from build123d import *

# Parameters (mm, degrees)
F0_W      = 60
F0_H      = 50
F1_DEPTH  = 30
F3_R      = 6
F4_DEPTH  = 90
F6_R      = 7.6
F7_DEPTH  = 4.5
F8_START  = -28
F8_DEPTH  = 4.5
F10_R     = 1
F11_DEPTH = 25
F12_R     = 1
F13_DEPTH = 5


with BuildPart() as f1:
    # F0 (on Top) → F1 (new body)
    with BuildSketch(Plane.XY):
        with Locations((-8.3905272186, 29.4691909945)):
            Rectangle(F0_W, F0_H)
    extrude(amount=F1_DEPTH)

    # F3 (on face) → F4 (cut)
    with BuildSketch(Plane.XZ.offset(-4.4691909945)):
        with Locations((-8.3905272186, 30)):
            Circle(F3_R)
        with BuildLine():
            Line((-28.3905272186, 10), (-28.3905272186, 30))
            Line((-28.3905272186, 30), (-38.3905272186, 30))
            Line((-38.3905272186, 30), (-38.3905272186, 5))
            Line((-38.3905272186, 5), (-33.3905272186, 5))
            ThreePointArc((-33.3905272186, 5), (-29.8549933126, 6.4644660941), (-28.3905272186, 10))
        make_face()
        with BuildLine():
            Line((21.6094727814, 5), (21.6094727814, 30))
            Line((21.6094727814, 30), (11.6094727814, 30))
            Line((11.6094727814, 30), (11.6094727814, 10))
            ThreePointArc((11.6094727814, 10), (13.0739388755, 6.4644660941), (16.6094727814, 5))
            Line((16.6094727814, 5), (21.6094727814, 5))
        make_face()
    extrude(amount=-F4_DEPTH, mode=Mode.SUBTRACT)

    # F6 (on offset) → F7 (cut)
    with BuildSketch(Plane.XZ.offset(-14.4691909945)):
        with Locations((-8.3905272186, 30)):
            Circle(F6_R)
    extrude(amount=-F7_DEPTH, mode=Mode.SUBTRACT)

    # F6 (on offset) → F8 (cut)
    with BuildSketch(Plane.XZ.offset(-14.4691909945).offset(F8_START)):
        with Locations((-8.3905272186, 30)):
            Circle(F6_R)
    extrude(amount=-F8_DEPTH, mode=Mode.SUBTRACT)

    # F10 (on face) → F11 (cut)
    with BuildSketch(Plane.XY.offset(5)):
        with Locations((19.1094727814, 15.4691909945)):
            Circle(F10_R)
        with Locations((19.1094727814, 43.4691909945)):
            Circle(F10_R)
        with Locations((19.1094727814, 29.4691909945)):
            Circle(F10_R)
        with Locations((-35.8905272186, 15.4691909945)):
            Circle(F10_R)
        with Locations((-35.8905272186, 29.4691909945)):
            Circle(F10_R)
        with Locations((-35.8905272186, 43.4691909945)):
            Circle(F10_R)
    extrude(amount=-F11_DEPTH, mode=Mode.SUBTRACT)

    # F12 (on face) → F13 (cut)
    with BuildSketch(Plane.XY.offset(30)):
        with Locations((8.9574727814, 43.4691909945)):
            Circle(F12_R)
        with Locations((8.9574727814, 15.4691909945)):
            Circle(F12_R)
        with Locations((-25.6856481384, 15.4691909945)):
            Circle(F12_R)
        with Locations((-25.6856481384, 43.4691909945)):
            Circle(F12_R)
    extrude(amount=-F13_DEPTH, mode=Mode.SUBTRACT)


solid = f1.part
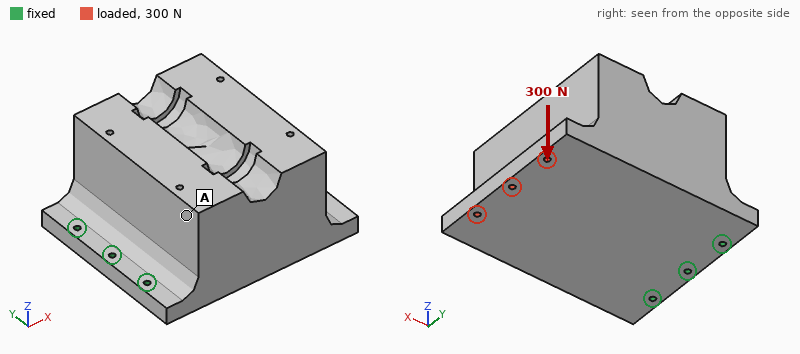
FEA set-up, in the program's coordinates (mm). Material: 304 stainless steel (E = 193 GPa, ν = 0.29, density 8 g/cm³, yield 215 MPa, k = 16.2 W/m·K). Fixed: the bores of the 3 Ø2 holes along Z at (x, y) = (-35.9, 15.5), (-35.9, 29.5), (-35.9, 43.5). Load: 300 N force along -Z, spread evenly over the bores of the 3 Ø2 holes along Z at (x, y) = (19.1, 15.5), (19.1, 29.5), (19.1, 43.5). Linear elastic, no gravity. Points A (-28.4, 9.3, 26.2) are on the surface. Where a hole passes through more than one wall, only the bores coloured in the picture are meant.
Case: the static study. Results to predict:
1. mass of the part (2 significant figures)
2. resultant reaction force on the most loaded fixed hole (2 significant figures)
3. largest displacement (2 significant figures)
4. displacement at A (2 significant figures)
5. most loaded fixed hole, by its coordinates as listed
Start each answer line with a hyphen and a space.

- 500 g
- 140 N
- 92 µm
- 39 µm
- (-35.9, 29.5)
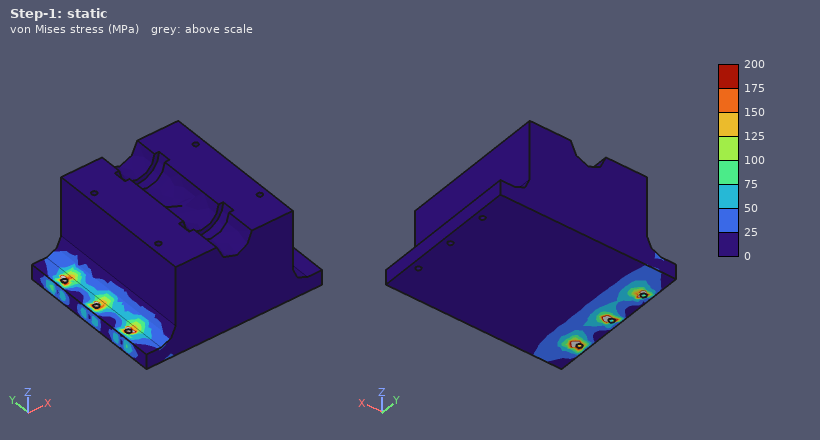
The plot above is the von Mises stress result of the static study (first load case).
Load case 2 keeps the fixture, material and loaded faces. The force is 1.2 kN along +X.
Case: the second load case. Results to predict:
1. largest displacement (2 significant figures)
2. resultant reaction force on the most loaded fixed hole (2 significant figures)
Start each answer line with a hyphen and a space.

- 3.9 µm
- 410 N
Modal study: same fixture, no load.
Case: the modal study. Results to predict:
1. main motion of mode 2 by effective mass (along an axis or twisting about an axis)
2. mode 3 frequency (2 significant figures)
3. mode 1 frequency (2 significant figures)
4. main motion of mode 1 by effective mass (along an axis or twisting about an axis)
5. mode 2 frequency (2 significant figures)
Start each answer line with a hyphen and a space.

- along Y
- 4000 Hz
- 700 Hz
- along Z
- 3200 Hz
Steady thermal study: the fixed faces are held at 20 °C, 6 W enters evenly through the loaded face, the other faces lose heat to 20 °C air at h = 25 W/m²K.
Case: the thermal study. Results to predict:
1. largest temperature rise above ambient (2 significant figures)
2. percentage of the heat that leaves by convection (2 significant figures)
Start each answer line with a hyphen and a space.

- 37 K
- 58 %
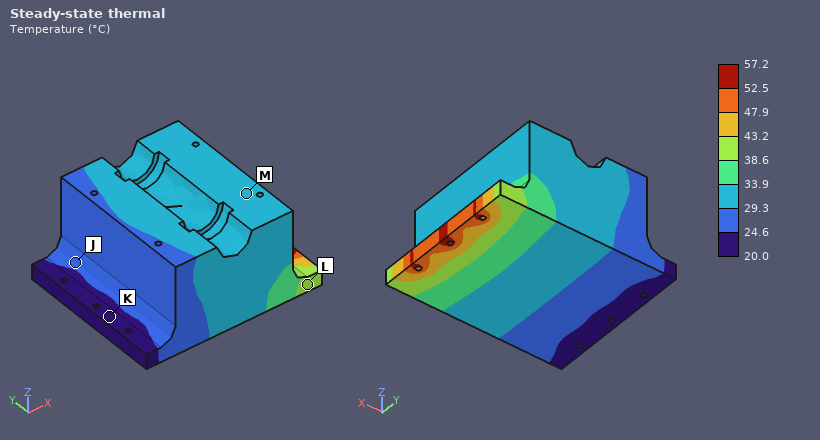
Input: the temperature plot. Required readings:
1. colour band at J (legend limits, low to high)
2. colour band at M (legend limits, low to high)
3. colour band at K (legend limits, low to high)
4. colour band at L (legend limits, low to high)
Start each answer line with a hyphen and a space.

- 24.6 to 29.3 °C
- 29.3 to 33.9 °C
- 20.0 to 24.6 °C
- 38.6 to 43.2 °C
